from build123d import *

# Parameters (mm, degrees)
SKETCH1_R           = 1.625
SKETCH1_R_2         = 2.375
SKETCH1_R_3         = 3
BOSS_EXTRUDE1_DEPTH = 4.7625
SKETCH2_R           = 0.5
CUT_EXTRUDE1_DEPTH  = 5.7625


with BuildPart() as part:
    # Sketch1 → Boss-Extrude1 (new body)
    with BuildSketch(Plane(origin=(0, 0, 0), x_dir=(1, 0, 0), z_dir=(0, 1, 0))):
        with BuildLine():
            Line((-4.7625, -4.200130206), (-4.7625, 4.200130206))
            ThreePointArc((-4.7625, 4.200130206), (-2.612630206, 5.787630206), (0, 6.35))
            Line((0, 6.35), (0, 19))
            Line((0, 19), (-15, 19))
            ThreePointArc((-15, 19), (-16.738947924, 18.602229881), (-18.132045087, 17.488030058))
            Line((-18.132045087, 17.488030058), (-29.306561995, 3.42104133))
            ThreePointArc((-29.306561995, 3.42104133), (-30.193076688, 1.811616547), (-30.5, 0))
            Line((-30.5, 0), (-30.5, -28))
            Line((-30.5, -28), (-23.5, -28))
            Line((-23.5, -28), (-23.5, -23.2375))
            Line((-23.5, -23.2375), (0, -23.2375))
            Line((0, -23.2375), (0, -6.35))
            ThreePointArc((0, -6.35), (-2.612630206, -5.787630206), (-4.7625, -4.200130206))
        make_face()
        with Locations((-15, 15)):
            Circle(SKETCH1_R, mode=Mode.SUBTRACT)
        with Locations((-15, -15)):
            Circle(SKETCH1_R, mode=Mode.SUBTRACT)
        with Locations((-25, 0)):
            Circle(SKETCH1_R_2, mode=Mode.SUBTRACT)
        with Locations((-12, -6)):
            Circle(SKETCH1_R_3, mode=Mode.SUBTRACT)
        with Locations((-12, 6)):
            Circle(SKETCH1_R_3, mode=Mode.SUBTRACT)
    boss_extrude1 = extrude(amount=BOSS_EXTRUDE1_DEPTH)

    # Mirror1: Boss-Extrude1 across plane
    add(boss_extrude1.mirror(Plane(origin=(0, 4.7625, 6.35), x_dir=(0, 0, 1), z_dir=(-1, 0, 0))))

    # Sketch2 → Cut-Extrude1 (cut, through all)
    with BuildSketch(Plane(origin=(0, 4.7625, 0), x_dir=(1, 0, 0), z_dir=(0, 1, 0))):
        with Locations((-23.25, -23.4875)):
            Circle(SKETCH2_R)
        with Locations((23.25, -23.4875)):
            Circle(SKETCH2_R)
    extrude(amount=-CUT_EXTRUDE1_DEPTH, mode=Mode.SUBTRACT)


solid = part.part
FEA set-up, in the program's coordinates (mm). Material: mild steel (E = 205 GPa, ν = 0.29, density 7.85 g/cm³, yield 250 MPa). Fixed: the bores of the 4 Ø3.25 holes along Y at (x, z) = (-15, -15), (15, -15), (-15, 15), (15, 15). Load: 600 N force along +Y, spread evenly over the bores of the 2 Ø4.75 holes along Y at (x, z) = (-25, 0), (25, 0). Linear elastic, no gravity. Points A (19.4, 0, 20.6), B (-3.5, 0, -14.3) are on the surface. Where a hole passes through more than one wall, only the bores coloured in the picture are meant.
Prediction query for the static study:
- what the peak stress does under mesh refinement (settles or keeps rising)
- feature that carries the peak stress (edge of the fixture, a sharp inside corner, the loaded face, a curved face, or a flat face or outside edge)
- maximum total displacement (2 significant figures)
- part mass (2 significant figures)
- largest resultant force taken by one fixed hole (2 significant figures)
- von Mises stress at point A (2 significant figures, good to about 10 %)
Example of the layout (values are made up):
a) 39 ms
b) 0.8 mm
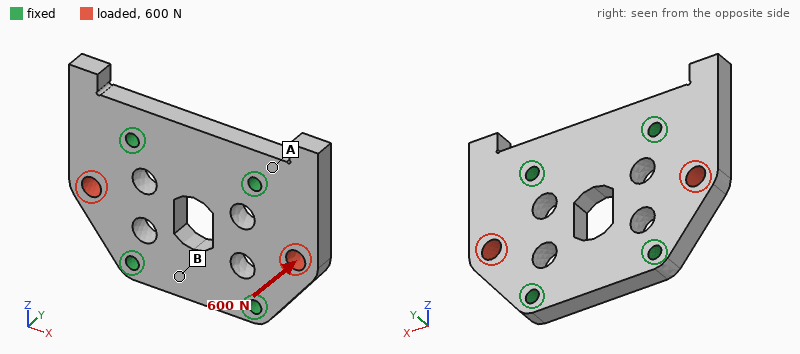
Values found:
a) keeps rising
b) edge of the fixture
c) 8.7 µm
d) 79 g
e) 150 N
f) 12 MPa
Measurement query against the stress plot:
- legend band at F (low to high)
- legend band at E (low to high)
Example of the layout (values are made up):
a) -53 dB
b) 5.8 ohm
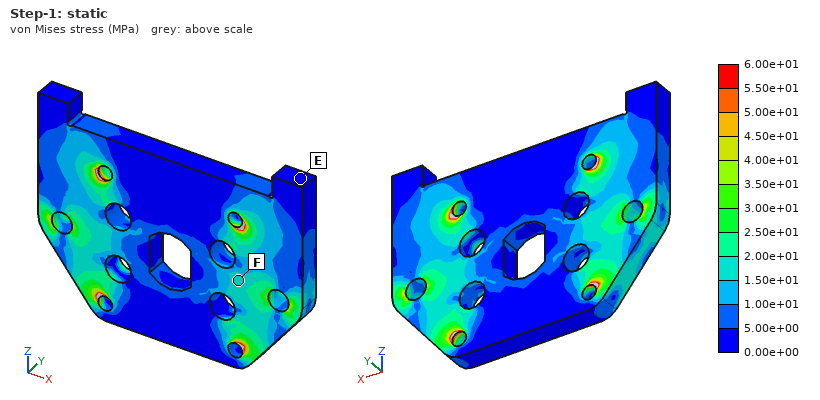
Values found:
a) 1.50e+01 to 2.00e+01 MPa
b) 0.00e+00 to 5.00e+00 MPa
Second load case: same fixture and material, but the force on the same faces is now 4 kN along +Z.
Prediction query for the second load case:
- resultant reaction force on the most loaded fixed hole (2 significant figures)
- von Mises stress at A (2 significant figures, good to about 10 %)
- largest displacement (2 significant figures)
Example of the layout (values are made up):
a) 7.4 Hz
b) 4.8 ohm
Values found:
a) 1.2 kN
b) 11 MPa
c) 3.4 µm
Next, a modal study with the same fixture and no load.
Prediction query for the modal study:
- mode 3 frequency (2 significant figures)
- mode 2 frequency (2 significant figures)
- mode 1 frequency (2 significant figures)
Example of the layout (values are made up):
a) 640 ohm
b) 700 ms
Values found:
a) 16 kHz
b) 12 kHz
c) 12 kHz
